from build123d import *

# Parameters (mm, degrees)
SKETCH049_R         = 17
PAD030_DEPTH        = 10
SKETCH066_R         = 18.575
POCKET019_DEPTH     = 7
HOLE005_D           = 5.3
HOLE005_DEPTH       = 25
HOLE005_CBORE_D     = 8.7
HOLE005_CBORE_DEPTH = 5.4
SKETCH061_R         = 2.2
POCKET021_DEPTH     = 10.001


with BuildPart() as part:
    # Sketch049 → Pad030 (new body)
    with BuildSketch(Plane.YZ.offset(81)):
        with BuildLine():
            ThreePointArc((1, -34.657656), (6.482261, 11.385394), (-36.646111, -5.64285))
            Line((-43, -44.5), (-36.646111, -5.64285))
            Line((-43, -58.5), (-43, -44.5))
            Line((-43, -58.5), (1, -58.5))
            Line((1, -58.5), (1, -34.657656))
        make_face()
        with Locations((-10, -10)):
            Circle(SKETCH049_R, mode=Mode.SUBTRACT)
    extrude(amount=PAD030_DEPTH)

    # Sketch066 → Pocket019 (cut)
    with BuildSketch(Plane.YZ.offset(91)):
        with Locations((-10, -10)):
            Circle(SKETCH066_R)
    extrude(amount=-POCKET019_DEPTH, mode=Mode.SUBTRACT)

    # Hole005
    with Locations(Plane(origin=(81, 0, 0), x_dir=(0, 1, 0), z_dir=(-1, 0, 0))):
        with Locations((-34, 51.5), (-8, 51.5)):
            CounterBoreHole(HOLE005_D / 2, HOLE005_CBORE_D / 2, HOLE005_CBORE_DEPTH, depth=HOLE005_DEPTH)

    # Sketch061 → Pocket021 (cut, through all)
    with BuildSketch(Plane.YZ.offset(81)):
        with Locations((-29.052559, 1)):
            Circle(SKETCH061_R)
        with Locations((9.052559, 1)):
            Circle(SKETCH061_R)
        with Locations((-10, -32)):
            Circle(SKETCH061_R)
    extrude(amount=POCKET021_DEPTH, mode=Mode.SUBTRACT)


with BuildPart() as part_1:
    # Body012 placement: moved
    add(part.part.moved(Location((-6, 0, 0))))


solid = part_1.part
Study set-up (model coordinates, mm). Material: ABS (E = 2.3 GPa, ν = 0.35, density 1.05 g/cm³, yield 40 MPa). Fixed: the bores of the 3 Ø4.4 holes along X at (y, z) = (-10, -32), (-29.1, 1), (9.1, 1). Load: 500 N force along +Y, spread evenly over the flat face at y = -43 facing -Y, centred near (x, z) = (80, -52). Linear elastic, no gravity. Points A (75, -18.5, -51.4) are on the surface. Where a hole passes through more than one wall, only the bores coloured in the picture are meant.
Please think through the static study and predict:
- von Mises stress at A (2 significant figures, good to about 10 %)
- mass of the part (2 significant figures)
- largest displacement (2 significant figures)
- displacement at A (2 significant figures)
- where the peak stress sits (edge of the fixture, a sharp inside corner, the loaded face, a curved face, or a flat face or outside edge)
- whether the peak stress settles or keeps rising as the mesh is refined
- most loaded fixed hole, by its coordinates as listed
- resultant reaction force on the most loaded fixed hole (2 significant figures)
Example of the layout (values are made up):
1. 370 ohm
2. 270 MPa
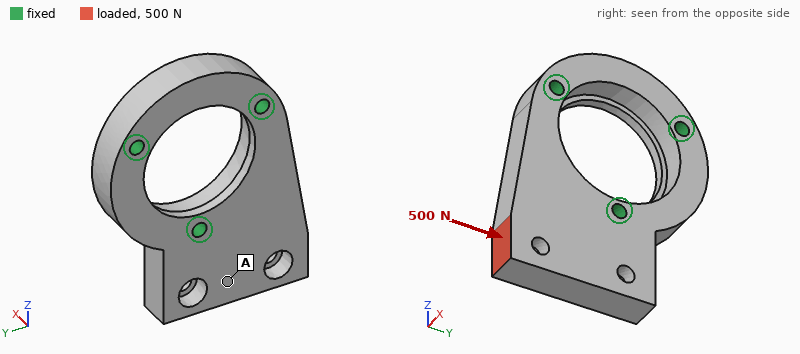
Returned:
1. 2.3 MPa
2. 24 g
3. 0.18 mm
4. 0.080 mm
5. edge of the fixture
6. keeps rising
7. (-10, -32)
8. 580 N
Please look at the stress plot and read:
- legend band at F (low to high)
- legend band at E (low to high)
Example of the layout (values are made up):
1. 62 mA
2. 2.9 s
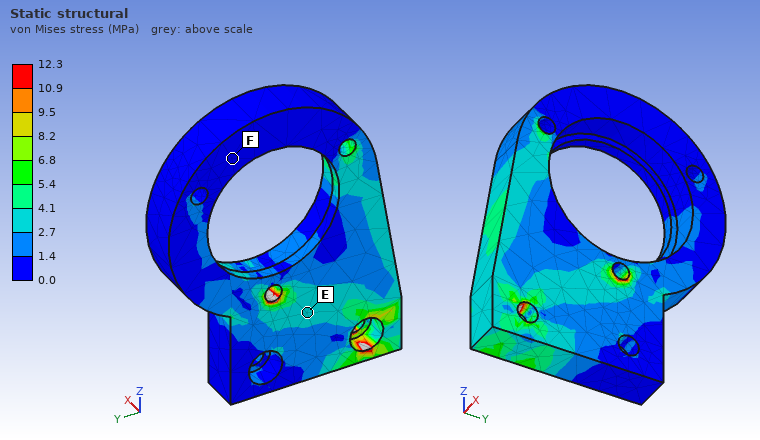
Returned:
1. 0.0 to 1.4 MPa
2. 2.7 to 4.1 MPa
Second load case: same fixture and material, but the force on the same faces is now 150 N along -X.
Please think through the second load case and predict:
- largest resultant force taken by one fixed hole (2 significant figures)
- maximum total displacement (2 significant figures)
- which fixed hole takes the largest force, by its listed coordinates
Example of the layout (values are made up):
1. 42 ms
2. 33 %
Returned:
1. 150 N
2. 0.75 mm
3. (-10, -32)
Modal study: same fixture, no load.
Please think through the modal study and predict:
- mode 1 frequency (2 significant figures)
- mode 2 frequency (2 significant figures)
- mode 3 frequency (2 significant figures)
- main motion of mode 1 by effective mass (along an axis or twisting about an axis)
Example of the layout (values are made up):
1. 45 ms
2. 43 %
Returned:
1. 1600 Hz
2. 3200 Hz
3. 3900 Hz
4. along X
